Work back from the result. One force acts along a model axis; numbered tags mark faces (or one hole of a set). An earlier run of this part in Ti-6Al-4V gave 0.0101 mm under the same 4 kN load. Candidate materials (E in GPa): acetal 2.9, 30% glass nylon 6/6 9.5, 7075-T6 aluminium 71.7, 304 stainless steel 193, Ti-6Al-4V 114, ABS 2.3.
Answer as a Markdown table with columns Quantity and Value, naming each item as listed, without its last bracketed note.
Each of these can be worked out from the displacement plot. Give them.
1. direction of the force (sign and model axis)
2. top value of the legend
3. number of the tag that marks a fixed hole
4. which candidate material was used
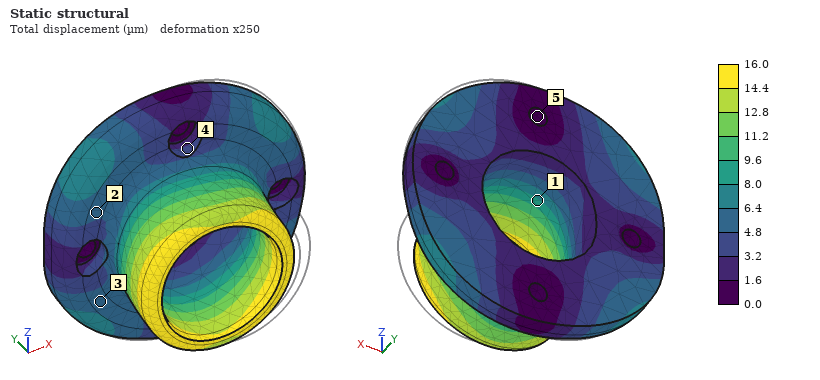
| Quantity | Value |
|---|---|
| direction of the force | -X |
| top value of the legend | 16.0 µm |
| number of the tag that marks a fixed hole | 5 |
| which candidate material was used | 7075-T6 aluminium |
